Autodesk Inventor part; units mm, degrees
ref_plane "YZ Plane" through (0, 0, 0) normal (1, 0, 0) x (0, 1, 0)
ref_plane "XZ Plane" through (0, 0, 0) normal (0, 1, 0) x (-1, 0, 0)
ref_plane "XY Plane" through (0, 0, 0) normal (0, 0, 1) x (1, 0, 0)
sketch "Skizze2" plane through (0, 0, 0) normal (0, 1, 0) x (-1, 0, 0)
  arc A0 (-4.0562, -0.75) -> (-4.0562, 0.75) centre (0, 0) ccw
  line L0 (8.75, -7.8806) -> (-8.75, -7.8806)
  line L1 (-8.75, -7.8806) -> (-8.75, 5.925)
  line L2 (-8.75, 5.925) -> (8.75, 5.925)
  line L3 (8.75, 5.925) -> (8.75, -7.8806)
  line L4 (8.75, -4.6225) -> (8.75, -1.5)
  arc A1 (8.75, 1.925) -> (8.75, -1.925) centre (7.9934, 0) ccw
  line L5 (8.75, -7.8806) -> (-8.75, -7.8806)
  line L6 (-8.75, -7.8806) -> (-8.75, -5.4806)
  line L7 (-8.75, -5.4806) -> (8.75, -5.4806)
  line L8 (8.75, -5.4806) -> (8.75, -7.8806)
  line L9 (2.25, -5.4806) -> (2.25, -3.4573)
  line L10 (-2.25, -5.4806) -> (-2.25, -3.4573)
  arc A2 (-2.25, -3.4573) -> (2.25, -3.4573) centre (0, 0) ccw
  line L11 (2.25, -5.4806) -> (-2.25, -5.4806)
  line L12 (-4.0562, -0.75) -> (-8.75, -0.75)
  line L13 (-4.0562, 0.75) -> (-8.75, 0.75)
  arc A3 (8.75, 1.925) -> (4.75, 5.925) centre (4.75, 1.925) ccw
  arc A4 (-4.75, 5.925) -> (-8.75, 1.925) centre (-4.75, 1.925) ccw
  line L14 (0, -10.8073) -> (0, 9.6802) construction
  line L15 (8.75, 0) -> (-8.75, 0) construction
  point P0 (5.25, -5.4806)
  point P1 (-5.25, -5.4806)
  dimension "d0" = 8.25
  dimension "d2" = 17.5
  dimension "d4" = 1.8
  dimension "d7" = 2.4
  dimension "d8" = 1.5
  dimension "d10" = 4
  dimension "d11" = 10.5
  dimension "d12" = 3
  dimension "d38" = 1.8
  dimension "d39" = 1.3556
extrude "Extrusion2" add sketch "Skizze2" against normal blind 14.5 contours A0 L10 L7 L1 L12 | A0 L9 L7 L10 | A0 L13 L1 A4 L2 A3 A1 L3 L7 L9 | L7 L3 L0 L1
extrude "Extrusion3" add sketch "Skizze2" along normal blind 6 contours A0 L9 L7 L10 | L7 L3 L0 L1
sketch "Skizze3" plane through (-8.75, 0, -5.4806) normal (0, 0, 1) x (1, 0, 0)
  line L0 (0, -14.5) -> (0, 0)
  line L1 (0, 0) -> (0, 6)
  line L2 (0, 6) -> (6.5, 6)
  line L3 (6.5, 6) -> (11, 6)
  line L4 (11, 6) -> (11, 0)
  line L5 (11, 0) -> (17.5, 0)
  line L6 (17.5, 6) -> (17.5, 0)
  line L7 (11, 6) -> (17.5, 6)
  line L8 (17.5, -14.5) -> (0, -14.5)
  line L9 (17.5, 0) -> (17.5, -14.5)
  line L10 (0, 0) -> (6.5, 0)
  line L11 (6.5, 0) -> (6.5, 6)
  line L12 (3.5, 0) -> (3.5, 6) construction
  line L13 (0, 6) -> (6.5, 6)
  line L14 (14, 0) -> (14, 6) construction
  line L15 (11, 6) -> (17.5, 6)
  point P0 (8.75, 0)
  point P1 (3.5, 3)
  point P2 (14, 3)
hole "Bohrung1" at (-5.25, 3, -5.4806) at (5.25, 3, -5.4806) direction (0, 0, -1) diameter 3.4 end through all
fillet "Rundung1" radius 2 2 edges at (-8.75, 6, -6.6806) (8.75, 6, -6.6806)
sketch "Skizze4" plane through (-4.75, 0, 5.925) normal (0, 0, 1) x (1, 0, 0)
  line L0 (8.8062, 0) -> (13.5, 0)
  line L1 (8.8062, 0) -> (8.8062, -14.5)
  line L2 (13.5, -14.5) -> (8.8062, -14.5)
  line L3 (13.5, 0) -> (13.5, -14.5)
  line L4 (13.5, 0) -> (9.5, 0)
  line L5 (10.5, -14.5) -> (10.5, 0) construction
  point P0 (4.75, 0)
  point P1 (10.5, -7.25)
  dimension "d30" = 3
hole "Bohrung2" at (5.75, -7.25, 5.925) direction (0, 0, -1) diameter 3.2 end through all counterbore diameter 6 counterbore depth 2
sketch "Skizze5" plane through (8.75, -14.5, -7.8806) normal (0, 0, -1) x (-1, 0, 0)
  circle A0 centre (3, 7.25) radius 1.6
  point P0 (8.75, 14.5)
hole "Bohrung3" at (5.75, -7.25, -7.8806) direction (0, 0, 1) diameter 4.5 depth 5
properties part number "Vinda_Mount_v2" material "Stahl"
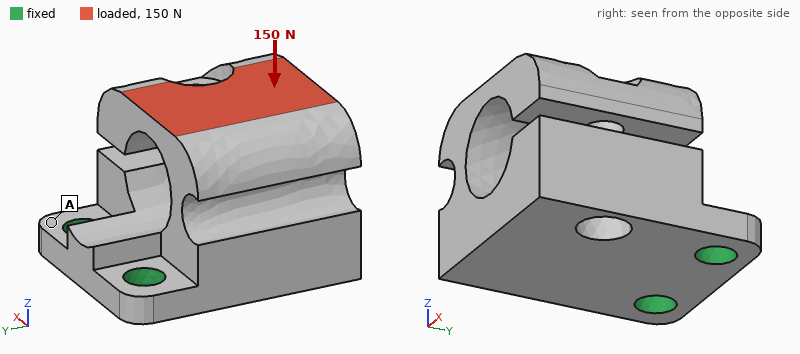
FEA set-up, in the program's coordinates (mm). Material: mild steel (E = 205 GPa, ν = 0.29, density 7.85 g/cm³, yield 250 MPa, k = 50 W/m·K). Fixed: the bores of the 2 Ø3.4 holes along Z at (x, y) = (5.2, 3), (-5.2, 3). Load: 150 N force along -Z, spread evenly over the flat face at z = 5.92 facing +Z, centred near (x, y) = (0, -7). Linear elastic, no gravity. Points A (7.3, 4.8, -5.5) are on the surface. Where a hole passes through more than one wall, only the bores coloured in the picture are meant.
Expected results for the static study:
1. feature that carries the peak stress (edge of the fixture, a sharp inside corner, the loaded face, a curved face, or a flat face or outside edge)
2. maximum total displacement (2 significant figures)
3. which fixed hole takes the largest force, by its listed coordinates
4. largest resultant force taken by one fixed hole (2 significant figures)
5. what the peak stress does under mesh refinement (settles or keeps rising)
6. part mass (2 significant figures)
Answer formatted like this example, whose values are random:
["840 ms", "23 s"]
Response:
["edge of the fixture", "39 µm", "(-5.2, 3)", "86 N", "keeps rising", "19 g"]
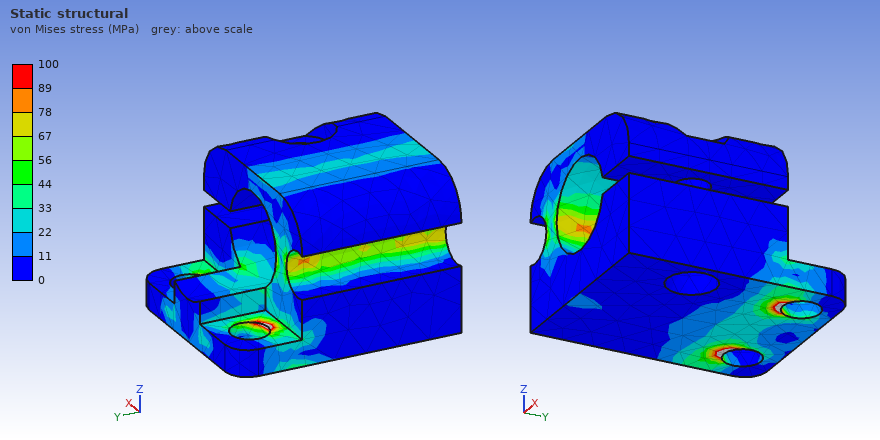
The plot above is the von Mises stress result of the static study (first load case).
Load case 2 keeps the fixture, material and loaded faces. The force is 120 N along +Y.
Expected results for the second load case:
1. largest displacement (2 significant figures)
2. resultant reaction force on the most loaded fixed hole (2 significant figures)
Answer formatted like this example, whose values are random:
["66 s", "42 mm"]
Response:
["23 µm", "61 N"]
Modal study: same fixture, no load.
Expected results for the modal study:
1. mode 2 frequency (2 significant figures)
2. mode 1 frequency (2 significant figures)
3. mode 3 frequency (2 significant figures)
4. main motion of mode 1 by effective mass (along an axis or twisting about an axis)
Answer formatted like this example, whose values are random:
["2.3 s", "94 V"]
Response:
["5100 Hz", "3900 Hz", "9900 Hz", "along Z"]
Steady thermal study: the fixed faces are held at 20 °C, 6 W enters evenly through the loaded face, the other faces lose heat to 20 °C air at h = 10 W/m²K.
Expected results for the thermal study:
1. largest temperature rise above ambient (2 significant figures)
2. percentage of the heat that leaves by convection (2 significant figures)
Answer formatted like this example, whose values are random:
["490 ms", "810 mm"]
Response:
["55 K", "7.7 %"]
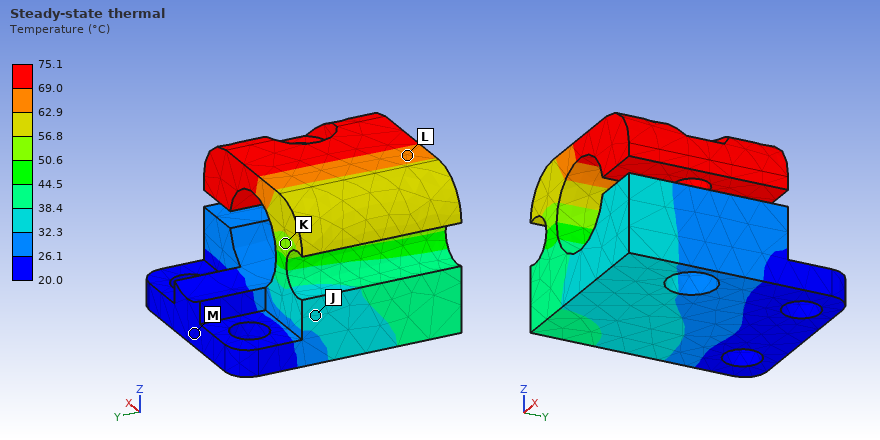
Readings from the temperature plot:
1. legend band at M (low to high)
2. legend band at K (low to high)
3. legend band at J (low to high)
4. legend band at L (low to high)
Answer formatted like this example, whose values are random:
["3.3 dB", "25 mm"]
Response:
["20.0 to 26.1 °C", "50.6 to 56.8 °C", "32.3 to 38.4 °C", "62.9 to 69.0 °C"]
